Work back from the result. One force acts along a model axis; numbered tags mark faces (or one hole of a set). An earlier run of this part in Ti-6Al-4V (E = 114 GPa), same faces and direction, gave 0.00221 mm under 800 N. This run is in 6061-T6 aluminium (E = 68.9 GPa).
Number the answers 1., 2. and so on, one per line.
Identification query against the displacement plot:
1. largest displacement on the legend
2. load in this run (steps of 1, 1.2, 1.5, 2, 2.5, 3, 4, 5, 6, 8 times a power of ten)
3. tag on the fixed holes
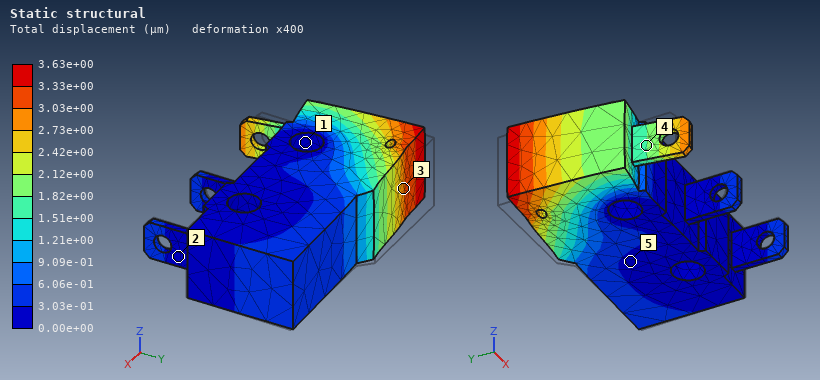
1. 3.63e+00 µm
2. 800 N
3. 1
